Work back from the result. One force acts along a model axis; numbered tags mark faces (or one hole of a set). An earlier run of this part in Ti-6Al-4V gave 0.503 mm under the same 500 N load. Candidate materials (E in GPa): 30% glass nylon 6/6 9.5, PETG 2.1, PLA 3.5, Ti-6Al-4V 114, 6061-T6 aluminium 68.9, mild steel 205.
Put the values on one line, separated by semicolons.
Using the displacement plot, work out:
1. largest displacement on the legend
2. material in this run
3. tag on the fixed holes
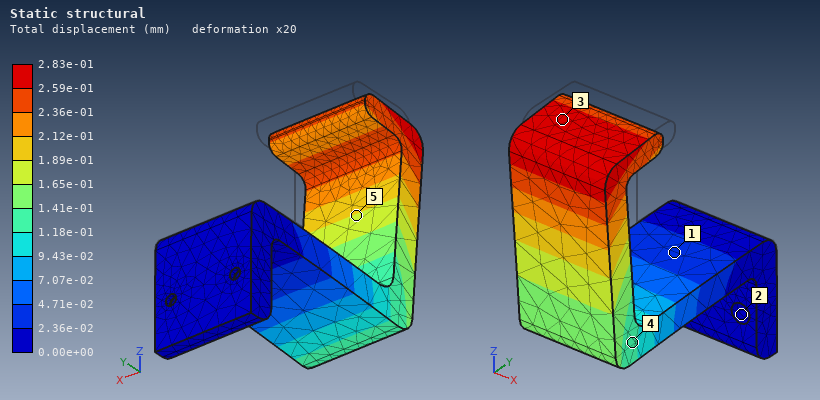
2.83e-01 mm; mild steel; 2
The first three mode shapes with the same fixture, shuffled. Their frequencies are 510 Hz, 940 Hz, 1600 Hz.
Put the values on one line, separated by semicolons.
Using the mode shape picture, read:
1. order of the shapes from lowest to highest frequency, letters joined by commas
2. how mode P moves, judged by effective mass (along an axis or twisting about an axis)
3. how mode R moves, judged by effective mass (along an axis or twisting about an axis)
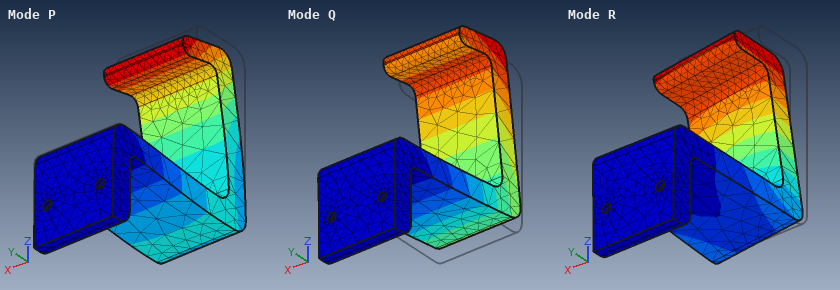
Q, R, P; along Z; along X
